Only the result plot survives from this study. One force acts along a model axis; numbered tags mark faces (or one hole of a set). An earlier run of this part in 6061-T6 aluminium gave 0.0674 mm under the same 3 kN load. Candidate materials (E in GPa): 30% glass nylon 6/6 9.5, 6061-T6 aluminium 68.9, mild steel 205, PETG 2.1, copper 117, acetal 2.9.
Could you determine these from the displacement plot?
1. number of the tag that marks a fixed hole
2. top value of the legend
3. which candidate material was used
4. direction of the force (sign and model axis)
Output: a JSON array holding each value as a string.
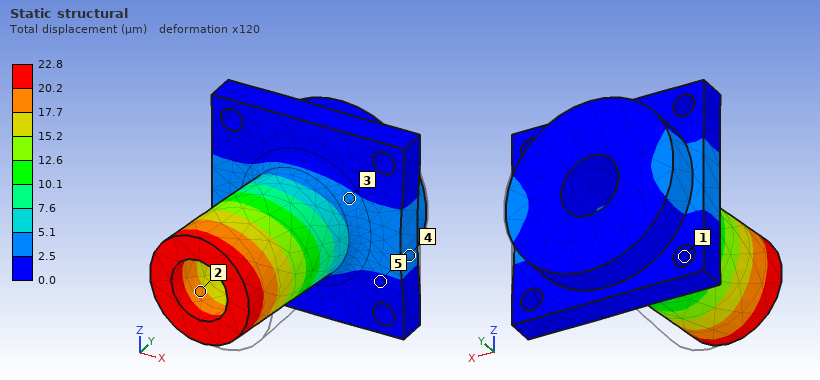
["1", "22.8 µm", "mild steel", "-X"]
